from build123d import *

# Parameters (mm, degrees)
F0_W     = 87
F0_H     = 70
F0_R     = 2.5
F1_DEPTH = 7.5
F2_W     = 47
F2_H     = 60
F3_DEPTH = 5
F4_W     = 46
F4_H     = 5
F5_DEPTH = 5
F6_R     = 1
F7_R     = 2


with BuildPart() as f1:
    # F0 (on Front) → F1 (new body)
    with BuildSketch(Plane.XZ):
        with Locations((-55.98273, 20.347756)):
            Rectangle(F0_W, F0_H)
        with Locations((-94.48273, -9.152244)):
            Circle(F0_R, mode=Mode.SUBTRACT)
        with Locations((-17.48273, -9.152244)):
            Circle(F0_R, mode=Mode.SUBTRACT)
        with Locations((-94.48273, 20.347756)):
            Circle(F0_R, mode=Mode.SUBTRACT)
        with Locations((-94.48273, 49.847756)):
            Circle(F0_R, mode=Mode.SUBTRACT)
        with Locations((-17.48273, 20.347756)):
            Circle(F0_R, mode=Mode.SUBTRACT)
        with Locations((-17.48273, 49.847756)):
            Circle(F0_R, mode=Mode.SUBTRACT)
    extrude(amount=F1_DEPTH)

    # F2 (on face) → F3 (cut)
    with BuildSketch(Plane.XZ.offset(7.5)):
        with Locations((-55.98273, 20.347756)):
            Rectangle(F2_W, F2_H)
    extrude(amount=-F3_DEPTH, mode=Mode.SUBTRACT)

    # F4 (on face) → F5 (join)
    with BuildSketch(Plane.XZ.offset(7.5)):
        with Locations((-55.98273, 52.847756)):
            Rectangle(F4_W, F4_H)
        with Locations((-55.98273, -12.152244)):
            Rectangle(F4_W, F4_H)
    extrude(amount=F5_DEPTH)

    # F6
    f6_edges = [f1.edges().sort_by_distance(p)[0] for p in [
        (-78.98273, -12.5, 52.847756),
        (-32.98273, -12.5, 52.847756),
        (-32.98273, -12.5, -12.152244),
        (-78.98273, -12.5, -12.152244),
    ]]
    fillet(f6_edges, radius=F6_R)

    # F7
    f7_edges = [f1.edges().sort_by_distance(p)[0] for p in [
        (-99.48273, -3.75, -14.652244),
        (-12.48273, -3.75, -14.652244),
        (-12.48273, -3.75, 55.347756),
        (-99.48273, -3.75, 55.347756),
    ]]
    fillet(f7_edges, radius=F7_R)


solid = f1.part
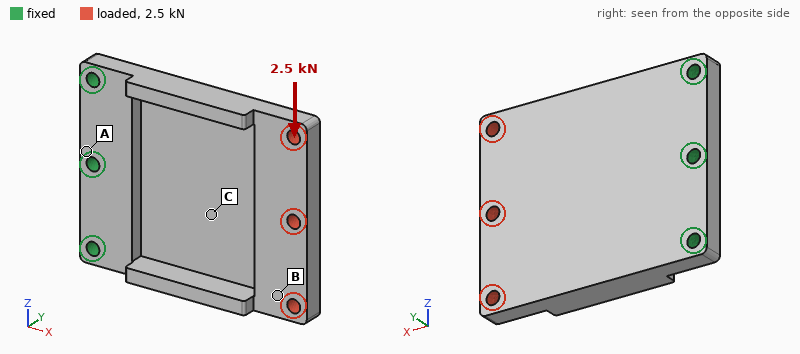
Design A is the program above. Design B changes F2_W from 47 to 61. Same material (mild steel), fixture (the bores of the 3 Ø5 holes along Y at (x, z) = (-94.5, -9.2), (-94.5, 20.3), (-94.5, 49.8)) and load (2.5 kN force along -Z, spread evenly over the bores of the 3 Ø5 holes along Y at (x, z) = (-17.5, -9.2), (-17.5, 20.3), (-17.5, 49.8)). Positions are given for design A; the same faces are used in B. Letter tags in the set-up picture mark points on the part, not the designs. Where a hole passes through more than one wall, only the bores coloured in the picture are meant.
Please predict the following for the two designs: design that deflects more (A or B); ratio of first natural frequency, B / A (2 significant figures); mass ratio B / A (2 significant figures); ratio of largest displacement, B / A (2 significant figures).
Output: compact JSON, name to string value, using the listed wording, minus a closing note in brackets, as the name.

{"design that deflects more": "B", "ratio of first natural frequency, B / A": "0.94", "mass ratio B / A": "0.87", "ratio of largest displacement, B / A": "1.5"}
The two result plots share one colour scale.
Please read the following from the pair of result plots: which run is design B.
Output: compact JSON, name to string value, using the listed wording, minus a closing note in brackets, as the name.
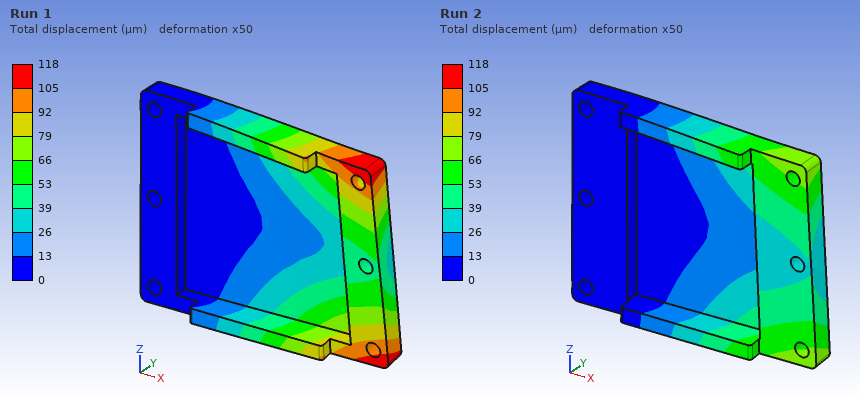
{"which run is design B": "Run 1"}
